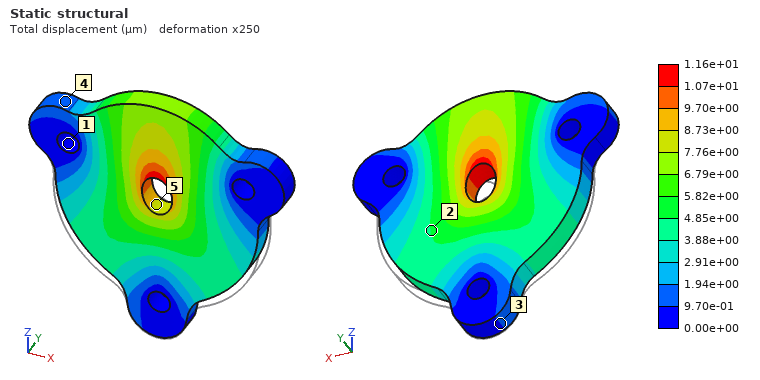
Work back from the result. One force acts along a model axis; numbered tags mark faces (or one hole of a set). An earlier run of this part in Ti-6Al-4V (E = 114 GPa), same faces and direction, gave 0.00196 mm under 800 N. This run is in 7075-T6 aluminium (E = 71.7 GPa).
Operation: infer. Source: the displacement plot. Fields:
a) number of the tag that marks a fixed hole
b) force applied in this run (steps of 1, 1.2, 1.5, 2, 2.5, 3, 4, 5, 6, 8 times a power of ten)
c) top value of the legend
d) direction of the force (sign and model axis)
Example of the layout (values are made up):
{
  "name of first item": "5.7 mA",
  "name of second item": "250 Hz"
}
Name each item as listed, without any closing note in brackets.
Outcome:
{
  "number of the tag that marks a fixed hole": "1",
  "force applied in this run": "3 kN",
  "top value of the legend": "1.16e+01 µm",
  "direction of the force": "+Z"
}
